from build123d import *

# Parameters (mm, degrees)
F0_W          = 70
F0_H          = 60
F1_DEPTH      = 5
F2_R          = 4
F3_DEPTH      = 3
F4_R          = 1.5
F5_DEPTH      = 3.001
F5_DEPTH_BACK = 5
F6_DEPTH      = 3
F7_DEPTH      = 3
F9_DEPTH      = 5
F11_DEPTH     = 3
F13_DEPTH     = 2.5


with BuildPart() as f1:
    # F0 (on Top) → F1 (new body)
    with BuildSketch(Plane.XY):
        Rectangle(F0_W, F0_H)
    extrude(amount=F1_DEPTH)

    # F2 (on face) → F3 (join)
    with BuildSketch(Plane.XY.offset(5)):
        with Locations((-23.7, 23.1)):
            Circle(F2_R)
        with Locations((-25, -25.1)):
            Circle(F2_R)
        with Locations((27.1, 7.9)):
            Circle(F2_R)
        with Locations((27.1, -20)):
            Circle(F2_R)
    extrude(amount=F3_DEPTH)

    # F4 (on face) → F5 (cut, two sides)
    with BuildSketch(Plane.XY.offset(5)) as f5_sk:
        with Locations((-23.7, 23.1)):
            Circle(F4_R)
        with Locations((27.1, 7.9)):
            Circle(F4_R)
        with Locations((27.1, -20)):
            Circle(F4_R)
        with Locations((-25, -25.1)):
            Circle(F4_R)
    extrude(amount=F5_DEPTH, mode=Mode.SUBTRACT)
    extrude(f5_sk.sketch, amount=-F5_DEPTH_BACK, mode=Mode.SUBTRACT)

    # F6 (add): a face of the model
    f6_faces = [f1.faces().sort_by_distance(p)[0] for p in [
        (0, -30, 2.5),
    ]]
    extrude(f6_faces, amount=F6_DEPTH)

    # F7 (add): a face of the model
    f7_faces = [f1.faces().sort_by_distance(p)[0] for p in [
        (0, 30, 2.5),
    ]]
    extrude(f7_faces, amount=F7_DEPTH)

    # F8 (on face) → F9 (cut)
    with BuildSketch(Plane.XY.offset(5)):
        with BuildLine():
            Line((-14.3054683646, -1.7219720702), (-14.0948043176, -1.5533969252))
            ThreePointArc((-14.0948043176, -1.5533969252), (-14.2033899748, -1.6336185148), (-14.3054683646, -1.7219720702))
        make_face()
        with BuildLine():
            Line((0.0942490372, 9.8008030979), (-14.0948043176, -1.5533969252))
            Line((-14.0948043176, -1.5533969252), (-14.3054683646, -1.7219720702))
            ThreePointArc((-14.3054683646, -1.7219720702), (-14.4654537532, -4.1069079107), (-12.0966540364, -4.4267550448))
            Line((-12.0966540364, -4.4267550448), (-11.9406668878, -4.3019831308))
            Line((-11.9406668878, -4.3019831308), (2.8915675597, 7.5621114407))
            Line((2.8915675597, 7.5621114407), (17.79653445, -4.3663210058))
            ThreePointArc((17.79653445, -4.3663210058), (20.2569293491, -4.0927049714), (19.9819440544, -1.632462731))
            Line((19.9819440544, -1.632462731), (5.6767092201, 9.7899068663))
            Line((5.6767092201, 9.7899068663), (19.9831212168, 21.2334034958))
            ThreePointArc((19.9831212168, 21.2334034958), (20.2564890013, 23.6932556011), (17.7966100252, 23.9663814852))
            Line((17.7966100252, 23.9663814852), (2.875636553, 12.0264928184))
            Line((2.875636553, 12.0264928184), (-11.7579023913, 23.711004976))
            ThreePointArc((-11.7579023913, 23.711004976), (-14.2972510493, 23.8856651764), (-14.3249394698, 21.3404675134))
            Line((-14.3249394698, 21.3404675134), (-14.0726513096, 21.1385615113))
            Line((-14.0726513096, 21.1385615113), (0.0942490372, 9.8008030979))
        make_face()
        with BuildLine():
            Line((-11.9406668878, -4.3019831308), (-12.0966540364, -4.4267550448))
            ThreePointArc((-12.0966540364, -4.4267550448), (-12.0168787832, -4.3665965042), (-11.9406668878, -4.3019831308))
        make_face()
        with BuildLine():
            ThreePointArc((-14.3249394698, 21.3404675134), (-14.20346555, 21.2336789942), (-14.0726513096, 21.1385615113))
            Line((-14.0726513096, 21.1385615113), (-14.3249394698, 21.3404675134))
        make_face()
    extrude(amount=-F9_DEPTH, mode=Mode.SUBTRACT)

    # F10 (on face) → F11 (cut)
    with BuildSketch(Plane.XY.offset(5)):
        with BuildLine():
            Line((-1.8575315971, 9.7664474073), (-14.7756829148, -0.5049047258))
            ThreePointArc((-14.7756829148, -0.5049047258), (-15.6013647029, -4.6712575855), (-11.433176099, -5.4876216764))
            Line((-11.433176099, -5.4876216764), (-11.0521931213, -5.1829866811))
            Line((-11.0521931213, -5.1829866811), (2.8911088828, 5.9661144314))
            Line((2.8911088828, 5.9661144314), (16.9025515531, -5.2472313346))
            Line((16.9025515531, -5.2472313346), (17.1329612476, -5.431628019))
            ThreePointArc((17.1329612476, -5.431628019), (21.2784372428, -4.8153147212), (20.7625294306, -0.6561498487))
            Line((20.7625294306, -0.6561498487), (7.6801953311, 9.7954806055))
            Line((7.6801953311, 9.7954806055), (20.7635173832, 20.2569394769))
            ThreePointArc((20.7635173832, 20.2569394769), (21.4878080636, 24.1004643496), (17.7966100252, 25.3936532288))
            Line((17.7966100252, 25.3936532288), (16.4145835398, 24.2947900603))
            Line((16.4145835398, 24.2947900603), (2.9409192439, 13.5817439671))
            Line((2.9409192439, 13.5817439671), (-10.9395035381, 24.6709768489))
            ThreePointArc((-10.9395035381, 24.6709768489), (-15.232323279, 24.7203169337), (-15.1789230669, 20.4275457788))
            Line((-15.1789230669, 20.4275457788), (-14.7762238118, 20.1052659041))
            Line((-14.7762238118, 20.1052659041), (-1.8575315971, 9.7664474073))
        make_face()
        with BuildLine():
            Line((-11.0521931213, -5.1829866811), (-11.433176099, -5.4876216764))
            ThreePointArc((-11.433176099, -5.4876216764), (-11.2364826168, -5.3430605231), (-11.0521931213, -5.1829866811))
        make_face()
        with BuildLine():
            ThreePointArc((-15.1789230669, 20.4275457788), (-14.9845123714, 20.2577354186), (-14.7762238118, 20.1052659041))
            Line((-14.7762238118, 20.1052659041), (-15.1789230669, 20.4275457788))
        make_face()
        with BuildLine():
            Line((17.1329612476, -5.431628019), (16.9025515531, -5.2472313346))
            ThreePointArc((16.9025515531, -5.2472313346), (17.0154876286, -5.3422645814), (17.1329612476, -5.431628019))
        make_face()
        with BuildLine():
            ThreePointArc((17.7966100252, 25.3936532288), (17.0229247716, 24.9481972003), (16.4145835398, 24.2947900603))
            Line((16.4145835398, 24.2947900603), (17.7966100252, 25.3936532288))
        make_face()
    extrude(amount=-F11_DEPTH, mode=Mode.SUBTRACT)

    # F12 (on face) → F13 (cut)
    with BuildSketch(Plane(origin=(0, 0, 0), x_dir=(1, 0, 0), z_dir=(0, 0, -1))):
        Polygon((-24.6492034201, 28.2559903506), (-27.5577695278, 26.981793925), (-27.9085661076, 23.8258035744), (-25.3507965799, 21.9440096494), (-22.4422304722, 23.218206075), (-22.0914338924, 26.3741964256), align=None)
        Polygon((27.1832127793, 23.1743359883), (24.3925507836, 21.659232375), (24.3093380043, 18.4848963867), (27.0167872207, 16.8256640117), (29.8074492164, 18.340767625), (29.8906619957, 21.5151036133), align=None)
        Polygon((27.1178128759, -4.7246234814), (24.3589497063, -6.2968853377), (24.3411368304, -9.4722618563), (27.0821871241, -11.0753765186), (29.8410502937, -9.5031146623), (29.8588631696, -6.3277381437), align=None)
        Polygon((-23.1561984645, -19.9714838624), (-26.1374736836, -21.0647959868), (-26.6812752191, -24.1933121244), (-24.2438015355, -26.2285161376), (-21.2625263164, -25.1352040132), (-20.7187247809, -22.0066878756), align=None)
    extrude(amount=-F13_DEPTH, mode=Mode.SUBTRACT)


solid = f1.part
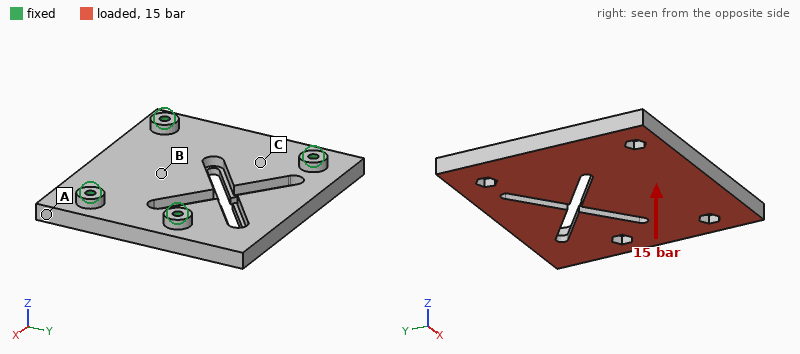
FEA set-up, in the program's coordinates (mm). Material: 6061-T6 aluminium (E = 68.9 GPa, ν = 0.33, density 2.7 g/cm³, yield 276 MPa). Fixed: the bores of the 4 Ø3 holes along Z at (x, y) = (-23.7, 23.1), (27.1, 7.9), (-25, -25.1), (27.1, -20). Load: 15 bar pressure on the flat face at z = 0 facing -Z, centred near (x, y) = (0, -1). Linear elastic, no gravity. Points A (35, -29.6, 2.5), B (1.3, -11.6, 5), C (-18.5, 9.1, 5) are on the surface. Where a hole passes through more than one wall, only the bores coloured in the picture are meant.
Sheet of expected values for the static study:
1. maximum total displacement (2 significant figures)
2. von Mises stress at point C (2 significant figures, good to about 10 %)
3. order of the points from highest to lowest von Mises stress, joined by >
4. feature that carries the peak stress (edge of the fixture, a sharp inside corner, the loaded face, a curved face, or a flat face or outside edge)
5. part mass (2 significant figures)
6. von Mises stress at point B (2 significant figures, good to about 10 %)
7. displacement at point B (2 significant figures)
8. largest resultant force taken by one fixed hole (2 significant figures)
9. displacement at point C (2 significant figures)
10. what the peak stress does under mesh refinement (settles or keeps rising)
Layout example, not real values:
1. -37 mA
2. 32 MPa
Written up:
1. 0.17 mm
2. 28 MPa
3. B > C > A
4. edge of the fixture
5. 57 g
6. 48 MPa
7. 0.094 mm
8. 2.0 kN
9. 0.058 mm
10. keeps rising
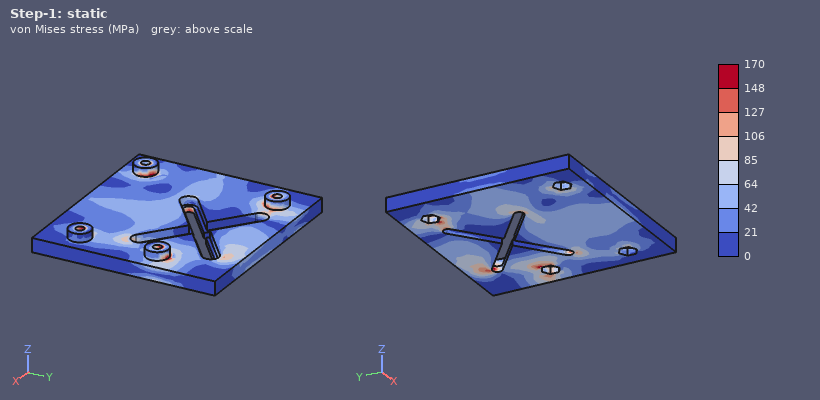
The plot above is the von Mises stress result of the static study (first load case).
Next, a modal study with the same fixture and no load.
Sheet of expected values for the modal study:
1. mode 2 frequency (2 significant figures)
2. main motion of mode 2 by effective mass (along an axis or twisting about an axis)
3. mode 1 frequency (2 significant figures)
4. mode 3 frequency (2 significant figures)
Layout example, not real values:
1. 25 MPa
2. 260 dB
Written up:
1. 5900 Hz
2. along Z
3. 4900 Hz
4. 7600 Hz
